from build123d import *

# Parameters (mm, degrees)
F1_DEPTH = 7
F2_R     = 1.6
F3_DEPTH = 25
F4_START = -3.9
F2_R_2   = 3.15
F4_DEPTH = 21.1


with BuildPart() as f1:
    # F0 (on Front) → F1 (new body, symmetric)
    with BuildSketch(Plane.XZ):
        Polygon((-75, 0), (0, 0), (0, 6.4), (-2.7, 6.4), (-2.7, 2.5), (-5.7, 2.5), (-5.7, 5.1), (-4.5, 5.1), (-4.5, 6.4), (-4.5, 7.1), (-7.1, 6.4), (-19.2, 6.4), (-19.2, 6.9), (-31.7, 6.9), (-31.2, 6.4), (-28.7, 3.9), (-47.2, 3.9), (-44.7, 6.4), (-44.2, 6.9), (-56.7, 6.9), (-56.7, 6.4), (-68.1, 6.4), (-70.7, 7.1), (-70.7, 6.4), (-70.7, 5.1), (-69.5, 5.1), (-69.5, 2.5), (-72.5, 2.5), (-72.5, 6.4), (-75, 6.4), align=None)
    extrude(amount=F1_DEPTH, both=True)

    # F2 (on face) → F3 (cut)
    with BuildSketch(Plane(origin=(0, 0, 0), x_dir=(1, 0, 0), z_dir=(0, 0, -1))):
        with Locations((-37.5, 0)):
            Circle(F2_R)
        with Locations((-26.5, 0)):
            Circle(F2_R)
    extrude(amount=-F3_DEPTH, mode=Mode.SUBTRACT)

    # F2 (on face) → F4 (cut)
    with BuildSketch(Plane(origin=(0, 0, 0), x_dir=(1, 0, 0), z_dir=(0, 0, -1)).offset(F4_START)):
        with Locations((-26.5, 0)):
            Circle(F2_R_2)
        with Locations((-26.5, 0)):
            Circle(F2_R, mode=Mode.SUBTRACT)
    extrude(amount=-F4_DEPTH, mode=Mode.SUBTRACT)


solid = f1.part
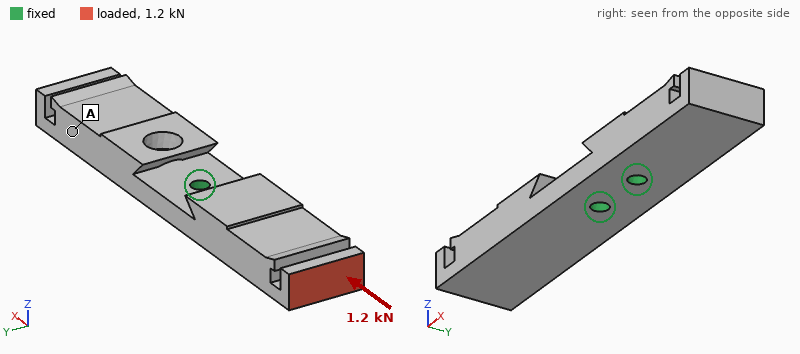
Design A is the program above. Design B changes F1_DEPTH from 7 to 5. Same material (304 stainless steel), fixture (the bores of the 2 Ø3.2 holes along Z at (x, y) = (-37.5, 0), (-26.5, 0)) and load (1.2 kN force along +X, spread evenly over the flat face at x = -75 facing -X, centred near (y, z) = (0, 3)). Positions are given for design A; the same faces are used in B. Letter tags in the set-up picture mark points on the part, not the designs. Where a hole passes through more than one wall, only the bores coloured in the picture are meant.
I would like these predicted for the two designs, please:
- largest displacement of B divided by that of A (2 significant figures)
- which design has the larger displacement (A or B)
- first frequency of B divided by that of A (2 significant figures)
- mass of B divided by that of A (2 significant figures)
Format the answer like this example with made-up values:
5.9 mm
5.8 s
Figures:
1.4
B
1.0
0.71
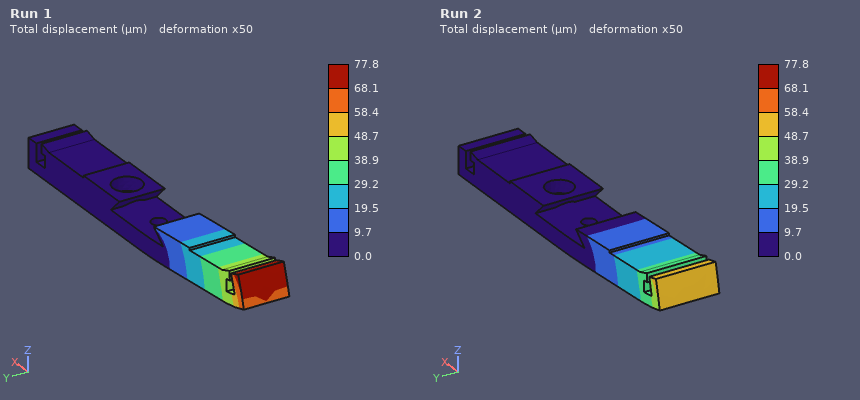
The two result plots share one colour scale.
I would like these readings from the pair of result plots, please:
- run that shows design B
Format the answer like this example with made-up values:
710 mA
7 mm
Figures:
Run 1
